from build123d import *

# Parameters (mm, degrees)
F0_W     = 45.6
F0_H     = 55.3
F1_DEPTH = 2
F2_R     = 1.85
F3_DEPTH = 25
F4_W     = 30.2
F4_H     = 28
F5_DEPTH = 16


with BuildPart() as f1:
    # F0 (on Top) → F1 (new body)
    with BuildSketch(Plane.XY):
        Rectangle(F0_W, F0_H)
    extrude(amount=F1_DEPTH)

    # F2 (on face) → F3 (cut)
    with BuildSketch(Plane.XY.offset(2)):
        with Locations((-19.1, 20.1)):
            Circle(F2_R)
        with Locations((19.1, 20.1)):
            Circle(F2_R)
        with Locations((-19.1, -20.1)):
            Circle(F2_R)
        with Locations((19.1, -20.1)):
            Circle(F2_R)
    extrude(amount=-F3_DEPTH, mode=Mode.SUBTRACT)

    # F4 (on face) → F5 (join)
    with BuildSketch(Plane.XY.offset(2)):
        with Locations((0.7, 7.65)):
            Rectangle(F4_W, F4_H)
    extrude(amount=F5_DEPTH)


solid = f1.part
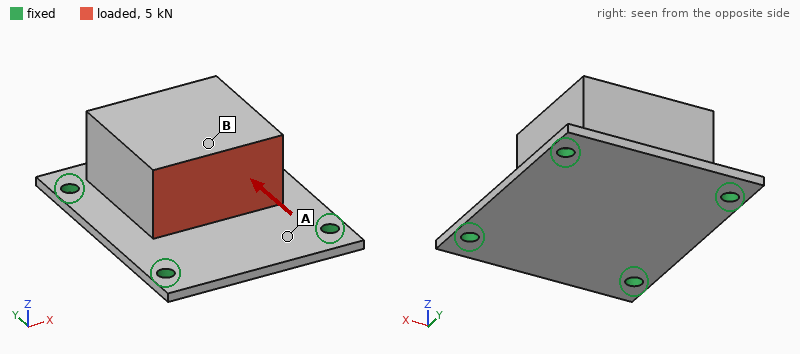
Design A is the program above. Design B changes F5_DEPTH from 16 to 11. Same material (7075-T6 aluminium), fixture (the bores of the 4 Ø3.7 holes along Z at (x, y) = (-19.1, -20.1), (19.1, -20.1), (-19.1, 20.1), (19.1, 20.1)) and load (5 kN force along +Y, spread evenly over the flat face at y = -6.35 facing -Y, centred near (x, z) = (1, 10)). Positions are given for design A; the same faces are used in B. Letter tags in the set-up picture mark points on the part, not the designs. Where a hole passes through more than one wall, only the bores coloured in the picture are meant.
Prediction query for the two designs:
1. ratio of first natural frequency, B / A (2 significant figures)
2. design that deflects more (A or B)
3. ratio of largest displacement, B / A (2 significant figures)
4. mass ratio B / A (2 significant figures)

1.2
A
0.66
0.77
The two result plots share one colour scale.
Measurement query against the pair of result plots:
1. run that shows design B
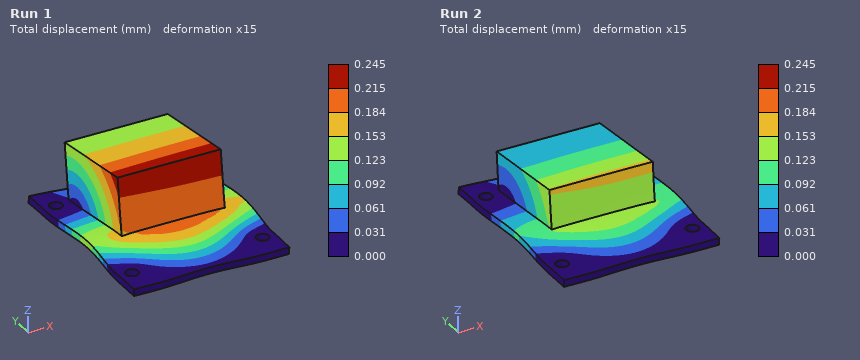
Run 2
